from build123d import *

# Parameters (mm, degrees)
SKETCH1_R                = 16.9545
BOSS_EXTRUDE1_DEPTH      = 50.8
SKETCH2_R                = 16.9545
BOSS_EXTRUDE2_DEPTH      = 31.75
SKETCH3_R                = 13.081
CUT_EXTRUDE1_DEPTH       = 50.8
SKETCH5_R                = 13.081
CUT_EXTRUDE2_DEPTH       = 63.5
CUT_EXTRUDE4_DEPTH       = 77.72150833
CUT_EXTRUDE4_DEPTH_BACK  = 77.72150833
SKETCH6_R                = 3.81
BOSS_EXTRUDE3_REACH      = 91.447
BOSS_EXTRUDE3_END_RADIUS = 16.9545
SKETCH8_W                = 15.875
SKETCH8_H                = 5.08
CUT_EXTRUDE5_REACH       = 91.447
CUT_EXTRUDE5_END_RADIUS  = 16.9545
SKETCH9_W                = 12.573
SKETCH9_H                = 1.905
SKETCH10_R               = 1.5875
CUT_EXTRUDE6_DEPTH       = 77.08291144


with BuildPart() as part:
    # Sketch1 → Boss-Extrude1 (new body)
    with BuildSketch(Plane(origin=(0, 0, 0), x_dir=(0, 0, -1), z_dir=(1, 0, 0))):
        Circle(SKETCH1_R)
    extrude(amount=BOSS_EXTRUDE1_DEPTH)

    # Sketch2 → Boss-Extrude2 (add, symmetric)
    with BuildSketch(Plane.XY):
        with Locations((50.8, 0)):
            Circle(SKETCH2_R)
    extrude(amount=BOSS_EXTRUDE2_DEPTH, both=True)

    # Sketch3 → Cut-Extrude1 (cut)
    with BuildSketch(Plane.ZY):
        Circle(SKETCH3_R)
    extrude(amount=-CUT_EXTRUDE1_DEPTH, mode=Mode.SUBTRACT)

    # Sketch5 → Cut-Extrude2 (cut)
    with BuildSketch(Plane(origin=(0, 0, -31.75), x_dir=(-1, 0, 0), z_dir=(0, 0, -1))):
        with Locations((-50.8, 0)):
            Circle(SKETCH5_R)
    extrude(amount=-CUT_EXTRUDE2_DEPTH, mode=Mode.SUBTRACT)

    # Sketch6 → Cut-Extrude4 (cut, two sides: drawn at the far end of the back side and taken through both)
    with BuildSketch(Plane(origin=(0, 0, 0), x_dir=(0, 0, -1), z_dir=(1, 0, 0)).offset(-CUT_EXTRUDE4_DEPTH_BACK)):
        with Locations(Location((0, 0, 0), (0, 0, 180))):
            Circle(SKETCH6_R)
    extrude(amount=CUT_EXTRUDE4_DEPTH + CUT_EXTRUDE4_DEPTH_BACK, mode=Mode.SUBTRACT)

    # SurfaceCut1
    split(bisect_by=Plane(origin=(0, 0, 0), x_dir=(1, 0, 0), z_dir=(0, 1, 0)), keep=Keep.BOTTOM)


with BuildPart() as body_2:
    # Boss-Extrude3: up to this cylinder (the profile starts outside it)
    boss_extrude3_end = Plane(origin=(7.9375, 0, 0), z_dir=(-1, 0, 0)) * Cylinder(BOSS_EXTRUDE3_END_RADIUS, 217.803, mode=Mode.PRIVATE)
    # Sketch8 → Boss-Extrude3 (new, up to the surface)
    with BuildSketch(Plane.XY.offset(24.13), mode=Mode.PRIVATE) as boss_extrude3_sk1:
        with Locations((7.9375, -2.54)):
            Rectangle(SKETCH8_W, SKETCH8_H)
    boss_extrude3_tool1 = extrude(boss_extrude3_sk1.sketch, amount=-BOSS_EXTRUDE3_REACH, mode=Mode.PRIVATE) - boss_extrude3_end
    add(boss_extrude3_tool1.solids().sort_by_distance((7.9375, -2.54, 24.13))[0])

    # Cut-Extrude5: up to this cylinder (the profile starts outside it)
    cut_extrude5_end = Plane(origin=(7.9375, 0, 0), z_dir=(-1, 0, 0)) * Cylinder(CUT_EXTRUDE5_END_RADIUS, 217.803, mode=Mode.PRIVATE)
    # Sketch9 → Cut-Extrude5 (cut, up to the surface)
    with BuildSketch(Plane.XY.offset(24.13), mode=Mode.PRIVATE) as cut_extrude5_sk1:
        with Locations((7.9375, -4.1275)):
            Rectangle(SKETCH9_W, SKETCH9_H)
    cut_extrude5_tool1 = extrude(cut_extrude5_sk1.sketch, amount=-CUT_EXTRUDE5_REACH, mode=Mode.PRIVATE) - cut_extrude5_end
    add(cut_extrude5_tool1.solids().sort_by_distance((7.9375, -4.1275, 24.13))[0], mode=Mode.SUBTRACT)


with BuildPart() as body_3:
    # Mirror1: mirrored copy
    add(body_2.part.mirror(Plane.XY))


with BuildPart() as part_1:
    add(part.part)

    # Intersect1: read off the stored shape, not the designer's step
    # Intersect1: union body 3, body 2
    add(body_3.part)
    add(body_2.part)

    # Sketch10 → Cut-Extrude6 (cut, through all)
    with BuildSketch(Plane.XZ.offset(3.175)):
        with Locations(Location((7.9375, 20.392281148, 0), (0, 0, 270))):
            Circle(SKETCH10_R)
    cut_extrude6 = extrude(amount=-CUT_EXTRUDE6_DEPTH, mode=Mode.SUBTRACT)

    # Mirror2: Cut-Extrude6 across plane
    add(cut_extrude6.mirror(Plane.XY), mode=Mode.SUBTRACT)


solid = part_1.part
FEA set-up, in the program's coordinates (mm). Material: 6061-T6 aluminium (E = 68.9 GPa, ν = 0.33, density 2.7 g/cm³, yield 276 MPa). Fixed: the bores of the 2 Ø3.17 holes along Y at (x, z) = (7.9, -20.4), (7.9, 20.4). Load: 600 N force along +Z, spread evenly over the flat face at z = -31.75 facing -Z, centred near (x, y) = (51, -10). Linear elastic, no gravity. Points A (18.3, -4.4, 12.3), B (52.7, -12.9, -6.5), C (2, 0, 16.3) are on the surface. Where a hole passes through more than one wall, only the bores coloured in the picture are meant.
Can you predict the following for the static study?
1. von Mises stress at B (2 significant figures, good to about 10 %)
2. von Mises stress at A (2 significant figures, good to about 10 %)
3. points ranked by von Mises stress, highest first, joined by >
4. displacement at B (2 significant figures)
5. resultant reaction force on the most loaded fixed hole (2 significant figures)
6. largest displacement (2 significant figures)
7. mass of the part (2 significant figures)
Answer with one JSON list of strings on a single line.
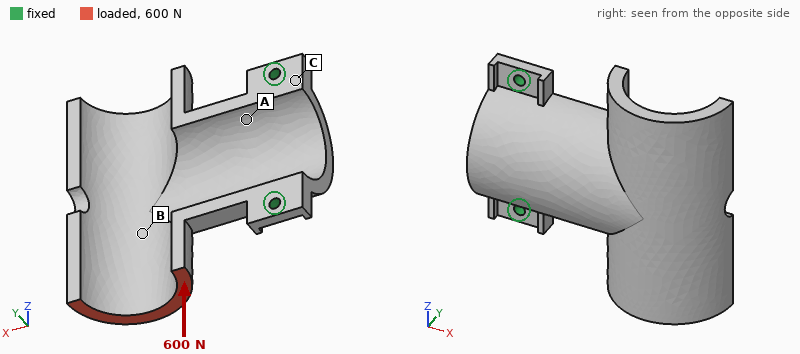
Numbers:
["17 MPa", "37 MPa", "A > B > C", "0.073 mm", "700 N", "0.22 mm", "49 g"]
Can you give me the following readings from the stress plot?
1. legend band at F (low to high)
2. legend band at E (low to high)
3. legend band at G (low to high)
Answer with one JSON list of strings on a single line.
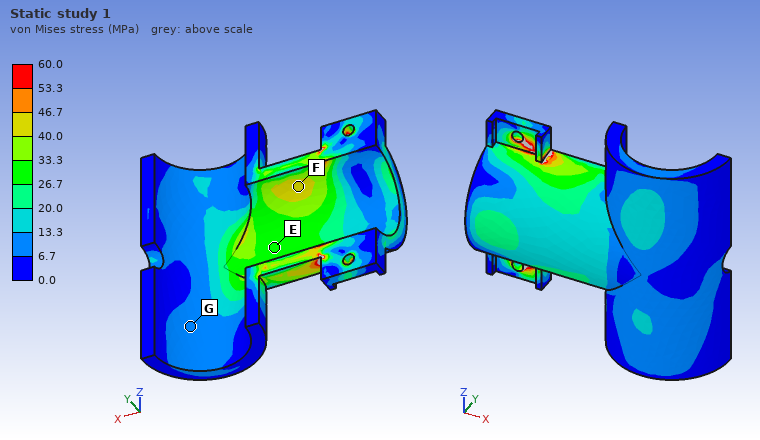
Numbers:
["40.0 to 46.7 MPa", "26.7 to 33.3 MPa", "6.7 to 13.3 MPa"]
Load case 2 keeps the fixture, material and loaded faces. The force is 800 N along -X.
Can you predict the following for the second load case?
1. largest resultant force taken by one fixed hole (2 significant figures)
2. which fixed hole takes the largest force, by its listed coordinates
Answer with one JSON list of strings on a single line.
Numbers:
["1.1 kN", "(7.9, -20.4)"]
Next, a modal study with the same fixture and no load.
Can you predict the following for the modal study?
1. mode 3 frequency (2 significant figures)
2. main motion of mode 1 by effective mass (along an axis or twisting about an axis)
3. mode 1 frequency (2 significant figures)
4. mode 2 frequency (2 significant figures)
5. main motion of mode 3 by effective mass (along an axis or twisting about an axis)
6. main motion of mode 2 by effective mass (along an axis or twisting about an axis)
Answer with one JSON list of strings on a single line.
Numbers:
["3600 Hz", "along Y", "790 Hz", "1500 Hz", "along Z", "along Z"]
